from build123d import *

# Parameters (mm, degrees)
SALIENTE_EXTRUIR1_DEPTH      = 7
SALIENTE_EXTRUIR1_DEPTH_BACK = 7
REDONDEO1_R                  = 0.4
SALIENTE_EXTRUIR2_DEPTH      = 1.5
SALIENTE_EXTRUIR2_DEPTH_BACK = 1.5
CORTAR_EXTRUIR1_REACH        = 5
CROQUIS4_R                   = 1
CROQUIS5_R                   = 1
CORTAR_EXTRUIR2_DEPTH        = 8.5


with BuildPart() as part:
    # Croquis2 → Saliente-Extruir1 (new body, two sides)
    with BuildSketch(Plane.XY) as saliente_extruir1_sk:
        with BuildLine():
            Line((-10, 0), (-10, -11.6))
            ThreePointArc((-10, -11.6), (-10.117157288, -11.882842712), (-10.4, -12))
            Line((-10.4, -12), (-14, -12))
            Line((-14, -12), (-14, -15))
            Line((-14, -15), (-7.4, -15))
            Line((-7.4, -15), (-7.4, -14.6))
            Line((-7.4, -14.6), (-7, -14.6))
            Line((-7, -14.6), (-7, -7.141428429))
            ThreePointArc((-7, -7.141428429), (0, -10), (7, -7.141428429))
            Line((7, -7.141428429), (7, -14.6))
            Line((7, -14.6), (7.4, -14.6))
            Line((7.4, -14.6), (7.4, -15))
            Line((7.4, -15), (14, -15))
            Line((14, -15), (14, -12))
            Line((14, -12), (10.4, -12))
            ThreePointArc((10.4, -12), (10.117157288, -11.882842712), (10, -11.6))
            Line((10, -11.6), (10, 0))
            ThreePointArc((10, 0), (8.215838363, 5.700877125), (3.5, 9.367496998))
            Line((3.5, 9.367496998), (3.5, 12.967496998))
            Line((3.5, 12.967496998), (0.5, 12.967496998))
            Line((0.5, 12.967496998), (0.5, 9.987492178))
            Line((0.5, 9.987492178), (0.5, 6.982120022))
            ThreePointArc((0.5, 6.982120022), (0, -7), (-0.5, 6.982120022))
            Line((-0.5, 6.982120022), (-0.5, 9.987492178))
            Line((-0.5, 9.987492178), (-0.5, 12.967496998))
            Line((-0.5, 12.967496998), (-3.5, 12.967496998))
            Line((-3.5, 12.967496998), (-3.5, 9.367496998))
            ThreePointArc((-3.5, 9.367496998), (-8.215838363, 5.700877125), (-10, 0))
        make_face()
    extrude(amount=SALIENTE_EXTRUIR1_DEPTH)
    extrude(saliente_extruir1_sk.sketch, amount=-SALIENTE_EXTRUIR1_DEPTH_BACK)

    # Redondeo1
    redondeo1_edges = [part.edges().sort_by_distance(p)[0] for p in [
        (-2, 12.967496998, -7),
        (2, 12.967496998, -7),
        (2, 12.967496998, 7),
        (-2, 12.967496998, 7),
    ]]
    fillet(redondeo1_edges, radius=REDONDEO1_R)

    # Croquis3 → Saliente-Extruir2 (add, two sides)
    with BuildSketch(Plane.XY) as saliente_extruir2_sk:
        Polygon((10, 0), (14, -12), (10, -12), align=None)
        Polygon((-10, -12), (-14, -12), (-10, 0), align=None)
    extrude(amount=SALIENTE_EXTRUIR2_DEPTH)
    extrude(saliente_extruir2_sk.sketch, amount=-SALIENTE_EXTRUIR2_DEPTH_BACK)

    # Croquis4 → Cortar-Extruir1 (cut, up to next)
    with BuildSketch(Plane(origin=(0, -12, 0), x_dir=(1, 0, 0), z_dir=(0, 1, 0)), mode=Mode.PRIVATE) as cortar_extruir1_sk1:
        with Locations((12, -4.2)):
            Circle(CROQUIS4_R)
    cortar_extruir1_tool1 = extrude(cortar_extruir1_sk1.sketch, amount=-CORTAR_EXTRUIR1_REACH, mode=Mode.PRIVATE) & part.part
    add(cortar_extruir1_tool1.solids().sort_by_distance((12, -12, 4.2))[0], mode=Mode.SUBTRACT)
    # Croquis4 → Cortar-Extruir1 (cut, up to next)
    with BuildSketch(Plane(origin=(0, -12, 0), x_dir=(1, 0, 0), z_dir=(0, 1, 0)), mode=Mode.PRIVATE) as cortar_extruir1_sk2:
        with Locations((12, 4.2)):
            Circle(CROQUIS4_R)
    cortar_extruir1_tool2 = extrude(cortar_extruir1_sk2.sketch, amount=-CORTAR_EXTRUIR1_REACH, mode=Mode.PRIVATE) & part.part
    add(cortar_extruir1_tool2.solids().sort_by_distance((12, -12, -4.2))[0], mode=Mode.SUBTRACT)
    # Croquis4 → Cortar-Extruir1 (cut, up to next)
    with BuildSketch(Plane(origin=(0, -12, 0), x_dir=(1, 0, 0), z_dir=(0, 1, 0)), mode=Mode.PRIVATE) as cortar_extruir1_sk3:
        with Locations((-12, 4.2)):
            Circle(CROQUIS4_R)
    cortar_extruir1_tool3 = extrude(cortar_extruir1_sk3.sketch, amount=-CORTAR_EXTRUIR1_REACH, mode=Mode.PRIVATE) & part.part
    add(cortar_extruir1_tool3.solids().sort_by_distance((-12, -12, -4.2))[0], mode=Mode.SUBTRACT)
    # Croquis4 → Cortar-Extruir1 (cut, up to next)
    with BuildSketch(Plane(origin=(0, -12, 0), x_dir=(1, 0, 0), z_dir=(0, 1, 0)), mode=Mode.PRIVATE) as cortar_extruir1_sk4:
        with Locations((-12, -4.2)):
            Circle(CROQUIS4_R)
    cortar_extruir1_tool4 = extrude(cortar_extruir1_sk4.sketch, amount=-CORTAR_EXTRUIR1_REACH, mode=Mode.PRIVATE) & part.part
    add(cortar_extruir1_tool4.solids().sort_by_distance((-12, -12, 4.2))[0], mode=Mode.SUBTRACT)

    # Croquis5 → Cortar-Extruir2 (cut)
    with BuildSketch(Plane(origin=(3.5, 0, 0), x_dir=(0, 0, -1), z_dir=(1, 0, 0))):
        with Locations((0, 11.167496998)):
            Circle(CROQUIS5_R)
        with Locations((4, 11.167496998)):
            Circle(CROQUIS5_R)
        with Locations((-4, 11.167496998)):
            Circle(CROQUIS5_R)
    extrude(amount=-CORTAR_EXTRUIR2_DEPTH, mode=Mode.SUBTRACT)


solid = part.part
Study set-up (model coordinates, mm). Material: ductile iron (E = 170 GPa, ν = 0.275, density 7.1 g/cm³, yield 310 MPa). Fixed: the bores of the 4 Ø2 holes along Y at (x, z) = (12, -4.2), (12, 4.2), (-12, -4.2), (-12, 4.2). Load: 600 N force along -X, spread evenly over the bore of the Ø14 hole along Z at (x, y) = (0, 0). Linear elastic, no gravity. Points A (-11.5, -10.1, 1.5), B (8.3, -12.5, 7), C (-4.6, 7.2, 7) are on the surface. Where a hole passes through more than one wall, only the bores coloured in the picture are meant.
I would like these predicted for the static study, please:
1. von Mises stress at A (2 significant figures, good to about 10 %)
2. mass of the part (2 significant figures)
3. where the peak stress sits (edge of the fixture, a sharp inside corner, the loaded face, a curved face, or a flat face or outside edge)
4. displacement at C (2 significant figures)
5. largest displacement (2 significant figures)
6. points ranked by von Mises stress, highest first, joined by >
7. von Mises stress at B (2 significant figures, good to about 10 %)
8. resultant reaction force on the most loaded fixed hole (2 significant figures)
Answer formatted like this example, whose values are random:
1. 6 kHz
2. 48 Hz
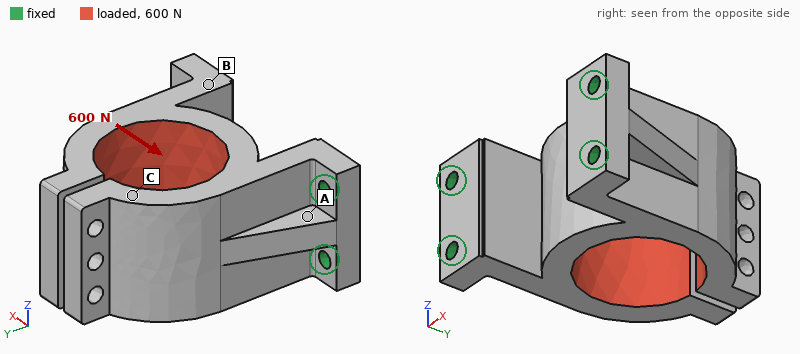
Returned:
1. 25 MPa
2. 26 g
3. a curved face
4. 21 µm
5. 31 µm
6. A > B > C
7. 14 MPa
8. 200 N
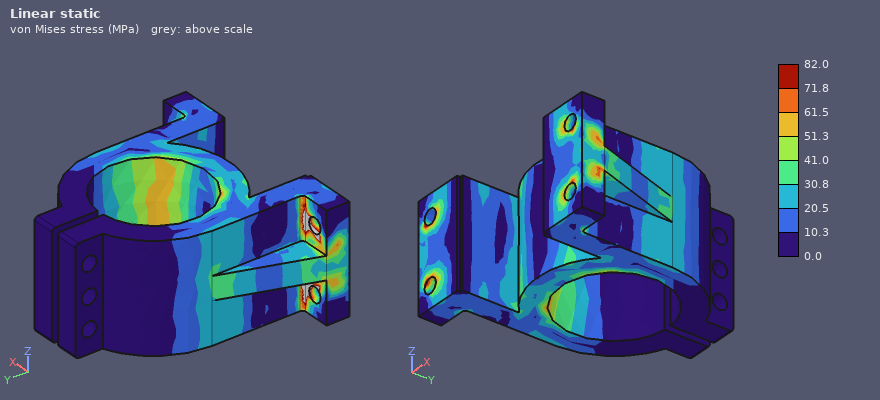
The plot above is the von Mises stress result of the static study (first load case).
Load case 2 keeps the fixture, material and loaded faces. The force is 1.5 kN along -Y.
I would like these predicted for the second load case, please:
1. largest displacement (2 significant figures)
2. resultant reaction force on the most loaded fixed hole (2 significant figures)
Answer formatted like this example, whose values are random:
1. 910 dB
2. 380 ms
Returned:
1. 56 µm
2. 440 N
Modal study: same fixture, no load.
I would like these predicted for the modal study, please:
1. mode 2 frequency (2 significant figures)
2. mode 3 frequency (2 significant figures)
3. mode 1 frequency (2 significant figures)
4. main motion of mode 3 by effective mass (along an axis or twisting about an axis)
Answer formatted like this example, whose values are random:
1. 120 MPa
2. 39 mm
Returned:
1. 5700 Hz
2. 8200 Hz
3. 5500 Hz
4. along Z
